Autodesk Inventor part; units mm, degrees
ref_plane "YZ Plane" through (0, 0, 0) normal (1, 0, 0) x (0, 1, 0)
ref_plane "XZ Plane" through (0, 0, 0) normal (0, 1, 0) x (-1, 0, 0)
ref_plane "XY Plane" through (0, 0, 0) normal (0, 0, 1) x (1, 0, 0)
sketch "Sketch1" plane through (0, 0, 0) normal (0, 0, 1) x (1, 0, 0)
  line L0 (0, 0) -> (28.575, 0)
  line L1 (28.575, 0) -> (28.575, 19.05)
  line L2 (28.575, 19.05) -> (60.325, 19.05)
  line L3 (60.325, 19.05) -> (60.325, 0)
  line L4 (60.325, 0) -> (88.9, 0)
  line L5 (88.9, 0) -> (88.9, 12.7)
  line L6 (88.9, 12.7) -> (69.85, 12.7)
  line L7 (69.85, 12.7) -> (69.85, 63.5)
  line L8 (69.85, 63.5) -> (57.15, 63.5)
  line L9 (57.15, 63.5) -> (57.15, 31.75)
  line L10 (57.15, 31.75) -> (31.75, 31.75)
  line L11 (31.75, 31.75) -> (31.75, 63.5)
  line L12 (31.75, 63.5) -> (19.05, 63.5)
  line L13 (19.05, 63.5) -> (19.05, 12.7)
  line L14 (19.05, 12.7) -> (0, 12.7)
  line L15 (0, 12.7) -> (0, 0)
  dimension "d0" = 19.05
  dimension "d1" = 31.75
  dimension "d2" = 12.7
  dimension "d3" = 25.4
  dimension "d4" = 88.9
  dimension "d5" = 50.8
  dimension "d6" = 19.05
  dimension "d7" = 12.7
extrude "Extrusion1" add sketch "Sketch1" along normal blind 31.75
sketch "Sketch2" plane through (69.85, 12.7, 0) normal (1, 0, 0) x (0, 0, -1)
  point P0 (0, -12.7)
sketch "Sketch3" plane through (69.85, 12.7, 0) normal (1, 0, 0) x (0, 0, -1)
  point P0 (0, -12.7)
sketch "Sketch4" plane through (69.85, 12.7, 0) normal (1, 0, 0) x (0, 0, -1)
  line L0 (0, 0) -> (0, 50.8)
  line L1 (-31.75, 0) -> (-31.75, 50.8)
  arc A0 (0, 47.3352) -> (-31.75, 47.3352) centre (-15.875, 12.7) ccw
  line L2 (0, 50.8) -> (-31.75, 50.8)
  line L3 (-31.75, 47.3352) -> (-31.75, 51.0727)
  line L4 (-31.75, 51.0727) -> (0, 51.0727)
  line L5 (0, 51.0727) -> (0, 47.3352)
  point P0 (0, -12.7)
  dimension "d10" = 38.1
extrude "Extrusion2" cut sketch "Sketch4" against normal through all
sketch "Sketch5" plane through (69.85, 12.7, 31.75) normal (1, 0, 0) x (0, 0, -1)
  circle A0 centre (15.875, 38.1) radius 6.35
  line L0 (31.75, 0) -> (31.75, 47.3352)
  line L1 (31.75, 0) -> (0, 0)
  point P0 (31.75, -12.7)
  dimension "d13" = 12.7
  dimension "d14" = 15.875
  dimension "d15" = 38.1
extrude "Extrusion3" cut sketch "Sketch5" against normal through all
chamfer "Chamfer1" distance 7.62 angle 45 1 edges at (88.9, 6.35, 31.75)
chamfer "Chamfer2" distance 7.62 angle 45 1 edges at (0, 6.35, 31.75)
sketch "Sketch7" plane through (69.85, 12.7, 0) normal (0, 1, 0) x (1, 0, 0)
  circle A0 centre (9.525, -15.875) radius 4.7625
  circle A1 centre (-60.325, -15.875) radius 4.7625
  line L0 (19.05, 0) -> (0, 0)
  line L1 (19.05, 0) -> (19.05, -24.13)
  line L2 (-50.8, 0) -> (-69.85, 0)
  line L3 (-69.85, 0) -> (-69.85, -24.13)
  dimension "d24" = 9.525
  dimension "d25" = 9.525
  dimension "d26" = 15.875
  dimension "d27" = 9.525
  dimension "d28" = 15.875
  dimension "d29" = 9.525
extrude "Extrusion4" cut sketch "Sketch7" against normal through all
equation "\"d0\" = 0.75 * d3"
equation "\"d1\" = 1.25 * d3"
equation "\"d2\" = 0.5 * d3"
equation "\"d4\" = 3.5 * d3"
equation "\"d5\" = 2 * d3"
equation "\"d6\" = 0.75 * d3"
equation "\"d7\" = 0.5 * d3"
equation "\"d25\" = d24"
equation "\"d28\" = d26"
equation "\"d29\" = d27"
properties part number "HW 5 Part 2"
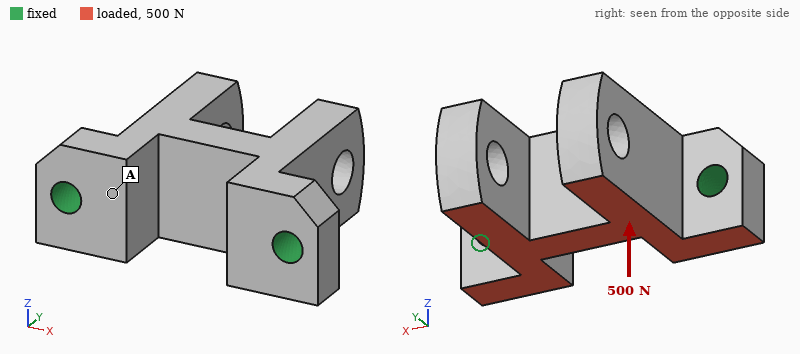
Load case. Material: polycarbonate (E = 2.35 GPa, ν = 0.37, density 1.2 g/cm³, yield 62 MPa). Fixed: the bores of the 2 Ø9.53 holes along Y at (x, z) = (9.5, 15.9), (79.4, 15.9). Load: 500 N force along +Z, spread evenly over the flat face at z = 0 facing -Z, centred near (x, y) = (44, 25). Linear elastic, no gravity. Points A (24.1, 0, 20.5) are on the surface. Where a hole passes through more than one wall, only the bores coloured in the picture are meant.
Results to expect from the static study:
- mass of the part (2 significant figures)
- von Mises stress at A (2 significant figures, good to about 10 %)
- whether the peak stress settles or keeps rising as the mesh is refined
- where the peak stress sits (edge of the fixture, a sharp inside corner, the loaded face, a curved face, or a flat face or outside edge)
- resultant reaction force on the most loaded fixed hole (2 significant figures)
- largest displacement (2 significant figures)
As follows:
80 g
1.5 MPa
keeps rising
edge of the fixture
250 N
0.27 mm
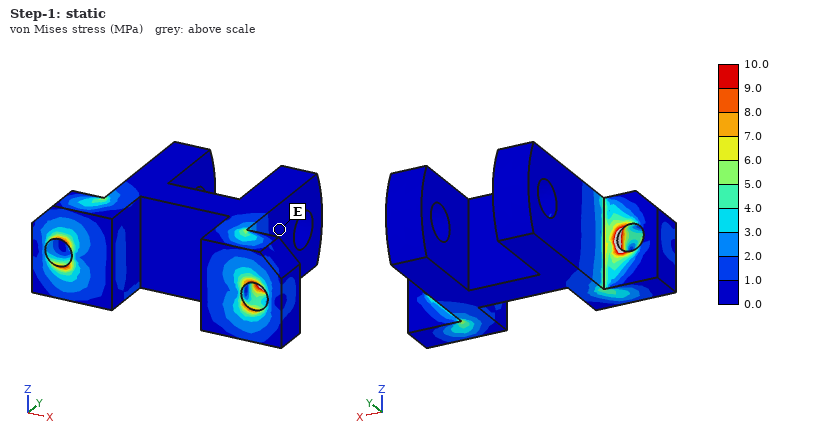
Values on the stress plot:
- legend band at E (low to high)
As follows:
0.0 to 1.0 MPa
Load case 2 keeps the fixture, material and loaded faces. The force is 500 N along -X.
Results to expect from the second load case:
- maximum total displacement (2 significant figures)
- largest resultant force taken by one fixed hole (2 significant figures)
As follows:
0.15 mm
300 N
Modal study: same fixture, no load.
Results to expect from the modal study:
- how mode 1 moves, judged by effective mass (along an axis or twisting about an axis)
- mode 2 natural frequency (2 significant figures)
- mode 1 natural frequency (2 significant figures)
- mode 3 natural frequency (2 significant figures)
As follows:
along Z
1500 Hz
940 Hz
1600 Hz
